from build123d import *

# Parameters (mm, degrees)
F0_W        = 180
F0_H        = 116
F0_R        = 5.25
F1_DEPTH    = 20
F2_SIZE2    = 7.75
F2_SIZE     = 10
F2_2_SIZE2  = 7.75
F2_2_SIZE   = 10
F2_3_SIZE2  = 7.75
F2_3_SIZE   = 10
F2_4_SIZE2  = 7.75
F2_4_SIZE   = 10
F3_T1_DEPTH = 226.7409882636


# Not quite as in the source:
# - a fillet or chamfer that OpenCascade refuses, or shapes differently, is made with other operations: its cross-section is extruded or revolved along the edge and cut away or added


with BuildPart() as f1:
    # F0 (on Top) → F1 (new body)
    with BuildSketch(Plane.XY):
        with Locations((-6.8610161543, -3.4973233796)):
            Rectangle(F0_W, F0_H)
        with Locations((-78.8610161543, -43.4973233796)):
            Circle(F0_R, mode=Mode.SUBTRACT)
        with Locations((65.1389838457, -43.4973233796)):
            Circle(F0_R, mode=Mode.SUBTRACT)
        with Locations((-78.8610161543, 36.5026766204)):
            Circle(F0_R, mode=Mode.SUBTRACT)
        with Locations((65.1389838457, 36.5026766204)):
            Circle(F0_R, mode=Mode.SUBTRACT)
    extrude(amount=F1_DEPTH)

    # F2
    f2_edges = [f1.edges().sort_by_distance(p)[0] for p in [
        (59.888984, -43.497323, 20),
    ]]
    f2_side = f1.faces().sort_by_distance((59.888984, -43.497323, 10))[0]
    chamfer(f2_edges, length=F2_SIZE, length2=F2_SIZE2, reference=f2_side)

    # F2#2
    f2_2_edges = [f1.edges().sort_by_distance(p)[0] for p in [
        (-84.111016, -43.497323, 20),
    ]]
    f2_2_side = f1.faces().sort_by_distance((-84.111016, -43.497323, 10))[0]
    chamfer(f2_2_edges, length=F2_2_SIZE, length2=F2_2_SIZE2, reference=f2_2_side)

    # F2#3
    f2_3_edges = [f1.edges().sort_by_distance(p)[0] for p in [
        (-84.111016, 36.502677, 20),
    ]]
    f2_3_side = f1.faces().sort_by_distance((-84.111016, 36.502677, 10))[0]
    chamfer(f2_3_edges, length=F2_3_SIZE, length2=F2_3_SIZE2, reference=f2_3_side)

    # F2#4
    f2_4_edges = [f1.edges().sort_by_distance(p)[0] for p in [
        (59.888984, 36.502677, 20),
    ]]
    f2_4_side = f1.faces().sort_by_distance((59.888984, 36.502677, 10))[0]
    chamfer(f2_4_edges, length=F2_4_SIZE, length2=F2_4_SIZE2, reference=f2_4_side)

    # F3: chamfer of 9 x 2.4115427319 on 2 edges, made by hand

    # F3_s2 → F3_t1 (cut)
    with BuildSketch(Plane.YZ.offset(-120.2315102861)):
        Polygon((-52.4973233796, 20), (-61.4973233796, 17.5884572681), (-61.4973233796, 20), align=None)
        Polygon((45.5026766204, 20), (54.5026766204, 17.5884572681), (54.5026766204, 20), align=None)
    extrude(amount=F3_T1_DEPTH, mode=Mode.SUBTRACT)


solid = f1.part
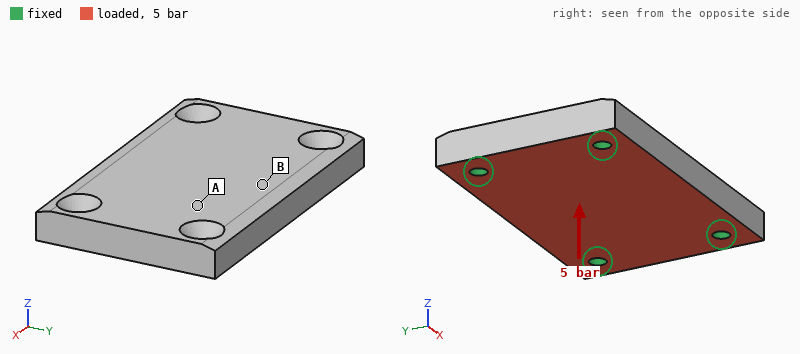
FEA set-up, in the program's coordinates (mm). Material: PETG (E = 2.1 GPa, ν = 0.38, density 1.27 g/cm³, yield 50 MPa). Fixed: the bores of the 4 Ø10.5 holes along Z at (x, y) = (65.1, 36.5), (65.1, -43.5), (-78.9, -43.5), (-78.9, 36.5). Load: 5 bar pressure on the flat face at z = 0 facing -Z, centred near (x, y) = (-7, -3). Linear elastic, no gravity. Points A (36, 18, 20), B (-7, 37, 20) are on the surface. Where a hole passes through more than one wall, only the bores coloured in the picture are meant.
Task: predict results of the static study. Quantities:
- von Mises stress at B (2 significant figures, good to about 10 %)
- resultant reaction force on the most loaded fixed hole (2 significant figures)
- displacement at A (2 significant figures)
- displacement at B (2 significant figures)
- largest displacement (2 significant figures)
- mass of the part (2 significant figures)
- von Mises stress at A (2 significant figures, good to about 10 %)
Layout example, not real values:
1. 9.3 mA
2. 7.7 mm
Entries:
1. 11 MPa
2. 3.0 kN
3. 0.54 mm
4. 0.89 mm
5. 0.95 mm
6. 510 g
7. 4.6 MPa
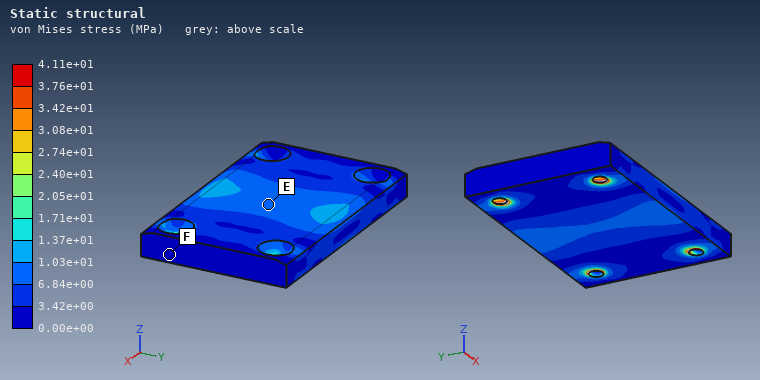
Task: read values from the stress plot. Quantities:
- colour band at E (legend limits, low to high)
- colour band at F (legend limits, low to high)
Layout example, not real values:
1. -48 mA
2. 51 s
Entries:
1. 6.84e+00 to 1.03e+01 MPa
2. 0.00e+00 to 3.42e+00 MPa
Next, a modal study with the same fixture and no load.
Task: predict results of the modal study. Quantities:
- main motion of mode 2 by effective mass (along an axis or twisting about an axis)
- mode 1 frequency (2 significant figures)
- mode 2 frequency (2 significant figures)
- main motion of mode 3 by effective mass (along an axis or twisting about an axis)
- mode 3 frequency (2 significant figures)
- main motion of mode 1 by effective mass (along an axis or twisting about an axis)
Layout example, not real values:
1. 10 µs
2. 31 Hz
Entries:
1. twisting about X
2. 830 Hz
3. 1200 Hz
4. along Y
5. 2100 Hz
6. along Z
